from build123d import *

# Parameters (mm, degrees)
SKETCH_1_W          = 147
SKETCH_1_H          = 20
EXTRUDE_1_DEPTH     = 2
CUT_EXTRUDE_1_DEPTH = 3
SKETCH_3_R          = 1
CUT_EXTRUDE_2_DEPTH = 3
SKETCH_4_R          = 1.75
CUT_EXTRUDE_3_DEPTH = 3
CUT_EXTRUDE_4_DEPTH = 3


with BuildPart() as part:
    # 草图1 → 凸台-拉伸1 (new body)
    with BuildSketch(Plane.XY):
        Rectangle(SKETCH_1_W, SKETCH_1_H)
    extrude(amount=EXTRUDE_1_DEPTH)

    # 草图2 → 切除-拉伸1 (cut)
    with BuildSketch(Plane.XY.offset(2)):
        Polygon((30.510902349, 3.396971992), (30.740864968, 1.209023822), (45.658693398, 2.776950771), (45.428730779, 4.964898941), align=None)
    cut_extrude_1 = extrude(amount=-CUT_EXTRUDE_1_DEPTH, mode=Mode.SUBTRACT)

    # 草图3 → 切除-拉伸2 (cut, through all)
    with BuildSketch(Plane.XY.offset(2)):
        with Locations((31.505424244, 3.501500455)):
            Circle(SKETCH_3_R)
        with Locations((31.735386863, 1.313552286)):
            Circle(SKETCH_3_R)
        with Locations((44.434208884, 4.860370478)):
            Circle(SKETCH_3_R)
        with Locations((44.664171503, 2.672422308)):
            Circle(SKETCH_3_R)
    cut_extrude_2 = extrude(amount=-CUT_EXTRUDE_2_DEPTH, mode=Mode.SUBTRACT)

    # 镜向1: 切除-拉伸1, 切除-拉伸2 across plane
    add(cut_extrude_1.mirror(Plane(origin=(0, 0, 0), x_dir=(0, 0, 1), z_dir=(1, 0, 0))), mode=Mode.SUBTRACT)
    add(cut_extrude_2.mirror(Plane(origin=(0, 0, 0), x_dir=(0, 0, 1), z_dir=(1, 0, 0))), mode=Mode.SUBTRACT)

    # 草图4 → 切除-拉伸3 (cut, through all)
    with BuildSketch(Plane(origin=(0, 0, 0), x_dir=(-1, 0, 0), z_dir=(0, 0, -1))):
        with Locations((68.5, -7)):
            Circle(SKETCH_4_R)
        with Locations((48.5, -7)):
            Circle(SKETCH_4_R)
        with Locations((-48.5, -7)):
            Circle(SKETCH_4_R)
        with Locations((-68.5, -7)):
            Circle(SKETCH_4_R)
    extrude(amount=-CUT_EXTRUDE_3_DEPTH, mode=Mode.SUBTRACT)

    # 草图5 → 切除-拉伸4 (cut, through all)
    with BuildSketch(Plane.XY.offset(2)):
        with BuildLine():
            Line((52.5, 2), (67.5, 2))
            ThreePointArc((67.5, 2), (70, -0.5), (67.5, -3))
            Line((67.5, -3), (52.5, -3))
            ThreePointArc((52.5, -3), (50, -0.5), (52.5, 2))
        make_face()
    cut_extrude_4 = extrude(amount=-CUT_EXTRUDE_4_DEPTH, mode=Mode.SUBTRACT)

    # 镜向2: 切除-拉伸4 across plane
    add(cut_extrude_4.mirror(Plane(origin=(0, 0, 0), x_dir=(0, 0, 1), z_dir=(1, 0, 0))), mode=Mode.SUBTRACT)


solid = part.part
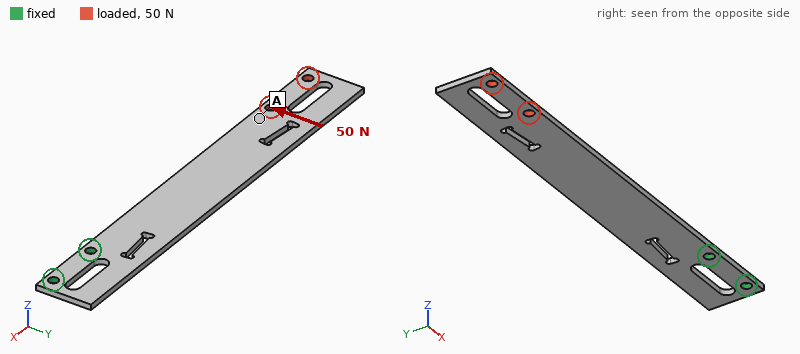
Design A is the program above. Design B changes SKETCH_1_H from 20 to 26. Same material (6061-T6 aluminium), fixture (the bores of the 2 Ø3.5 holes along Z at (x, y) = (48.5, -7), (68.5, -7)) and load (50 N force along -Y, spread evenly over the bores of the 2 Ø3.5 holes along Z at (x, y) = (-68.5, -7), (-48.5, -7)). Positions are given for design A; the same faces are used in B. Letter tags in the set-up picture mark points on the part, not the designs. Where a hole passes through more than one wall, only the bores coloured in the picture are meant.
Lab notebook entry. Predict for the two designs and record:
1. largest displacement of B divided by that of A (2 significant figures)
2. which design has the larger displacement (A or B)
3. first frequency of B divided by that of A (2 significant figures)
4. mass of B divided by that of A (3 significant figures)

0.53
A
0.99
1.33
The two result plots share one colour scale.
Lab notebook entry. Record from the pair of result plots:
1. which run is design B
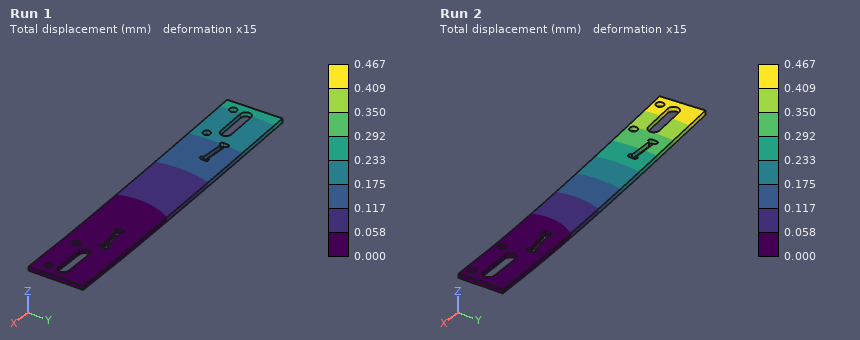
Run 1
